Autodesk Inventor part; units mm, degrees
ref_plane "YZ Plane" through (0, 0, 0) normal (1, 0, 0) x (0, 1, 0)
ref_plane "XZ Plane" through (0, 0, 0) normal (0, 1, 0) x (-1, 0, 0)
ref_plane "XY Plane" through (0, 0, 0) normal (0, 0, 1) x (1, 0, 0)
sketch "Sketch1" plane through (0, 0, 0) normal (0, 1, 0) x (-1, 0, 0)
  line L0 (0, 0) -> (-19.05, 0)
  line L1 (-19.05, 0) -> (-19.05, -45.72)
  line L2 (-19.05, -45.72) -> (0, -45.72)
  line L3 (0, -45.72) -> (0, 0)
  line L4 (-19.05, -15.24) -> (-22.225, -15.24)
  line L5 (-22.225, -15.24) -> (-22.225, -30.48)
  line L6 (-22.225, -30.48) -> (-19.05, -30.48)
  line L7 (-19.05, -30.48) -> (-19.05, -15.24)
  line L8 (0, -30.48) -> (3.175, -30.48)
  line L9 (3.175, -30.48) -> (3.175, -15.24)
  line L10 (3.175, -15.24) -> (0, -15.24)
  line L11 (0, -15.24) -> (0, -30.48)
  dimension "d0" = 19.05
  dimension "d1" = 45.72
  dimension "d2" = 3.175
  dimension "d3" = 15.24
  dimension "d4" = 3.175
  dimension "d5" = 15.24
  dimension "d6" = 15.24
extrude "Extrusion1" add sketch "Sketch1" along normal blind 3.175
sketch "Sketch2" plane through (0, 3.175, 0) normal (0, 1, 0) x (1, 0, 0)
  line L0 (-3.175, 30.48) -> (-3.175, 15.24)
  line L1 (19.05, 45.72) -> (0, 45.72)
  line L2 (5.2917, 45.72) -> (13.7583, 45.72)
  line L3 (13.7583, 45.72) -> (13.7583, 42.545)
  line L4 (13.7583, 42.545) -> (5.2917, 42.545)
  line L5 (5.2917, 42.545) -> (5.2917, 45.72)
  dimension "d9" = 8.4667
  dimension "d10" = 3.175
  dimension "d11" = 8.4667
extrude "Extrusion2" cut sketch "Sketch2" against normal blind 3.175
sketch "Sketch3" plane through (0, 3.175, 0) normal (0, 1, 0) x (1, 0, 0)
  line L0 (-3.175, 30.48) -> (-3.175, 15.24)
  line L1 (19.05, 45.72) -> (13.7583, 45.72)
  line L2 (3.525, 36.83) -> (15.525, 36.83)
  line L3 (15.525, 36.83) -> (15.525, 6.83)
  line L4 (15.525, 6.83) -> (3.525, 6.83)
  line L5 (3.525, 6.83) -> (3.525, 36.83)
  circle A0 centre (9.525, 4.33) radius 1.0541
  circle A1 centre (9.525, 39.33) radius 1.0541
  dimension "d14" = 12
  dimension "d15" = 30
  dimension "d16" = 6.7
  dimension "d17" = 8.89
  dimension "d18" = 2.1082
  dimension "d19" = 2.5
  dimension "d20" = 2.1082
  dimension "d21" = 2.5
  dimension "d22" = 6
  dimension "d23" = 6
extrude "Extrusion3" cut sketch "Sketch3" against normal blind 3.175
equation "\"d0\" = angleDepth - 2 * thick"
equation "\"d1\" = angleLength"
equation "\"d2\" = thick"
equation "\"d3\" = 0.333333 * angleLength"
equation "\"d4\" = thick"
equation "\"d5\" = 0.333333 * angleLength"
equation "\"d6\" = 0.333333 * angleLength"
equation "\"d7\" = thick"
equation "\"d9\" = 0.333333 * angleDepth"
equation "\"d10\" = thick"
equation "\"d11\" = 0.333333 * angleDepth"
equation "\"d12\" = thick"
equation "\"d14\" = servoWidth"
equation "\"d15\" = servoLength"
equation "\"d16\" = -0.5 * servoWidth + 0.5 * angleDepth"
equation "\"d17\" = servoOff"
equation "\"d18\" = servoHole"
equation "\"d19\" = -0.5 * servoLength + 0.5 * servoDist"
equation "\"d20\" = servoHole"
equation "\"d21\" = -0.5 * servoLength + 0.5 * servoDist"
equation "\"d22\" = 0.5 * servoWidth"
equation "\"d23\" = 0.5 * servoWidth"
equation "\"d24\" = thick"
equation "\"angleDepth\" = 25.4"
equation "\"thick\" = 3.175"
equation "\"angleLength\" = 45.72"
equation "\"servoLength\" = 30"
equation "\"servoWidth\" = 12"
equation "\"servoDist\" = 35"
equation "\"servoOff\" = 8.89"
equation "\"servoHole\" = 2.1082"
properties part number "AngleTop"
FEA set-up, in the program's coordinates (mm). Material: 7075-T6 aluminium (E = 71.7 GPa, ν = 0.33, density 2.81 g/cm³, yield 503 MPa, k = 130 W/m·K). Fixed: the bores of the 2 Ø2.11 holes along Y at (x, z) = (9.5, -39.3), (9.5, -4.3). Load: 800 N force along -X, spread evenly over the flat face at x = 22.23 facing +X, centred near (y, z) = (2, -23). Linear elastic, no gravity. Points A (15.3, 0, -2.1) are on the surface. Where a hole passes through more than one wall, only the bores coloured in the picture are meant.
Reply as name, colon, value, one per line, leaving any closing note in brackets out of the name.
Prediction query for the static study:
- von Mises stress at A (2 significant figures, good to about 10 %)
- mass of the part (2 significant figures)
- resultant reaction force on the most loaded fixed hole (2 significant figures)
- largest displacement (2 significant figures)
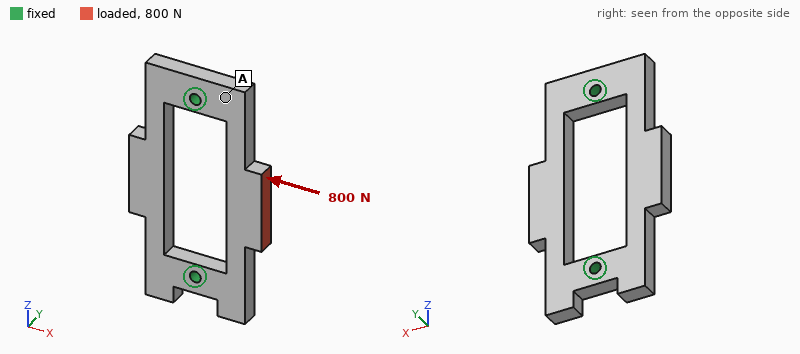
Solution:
von Mises stress at A: 26 MPa
mass of the part: 5.1 g
resultant reaction force on the most loaded fixed hole: 570 N
largest displacement: 87 µm
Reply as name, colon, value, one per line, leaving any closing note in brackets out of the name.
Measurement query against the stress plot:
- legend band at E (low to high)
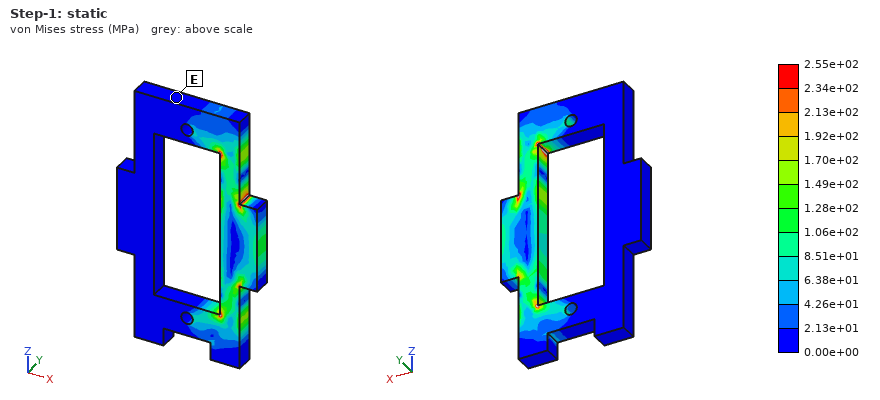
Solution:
legend band at E: 0.00e+00 to 2.13e+01 MPa
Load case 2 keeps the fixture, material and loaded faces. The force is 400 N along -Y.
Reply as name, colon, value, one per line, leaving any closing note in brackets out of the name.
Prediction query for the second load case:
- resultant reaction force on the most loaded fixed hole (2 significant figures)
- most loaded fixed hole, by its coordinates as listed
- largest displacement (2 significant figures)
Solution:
resultant reaction force on the most loaded fixed hole: 210 N
most loaded fixed hole, by its coordinates as listed: (9.5, -39.3)
largest displacement: 0.35 mm
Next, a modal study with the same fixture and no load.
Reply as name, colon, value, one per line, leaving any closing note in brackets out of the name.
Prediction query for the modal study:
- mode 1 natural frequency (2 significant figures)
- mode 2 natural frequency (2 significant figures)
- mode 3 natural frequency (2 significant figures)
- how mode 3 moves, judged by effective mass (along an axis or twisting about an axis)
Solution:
mode 1 natural frequency: 7100 Hz
mode 2 natural frequency: 7100 Hz
mode 3 natural frequency: 15 kHz
how mode 3 moves, judged by effective mass: along X
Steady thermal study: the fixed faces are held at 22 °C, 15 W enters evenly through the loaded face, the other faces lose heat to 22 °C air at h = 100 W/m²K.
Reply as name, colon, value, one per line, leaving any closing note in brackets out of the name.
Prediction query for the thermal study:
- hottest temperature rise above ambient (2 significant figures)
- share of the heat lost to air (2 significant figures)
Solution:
hottest temperature rise above ambient: 75 K
share of the heat lost to air: 20 %
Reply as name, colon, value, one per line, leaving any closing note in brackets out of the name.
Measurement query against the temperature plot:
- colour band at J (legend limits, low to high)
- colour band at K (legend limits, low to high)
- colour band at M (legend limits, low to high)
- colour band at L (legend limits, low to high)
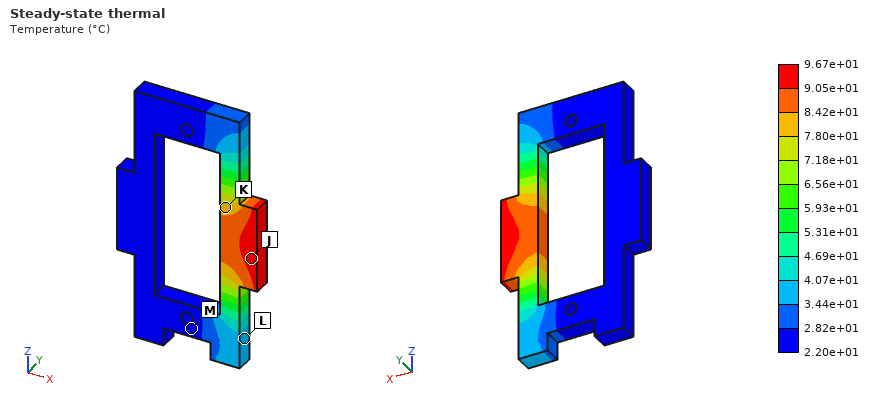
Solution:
colour band at J: 9.05e+01 to 9.67e+01 °C
colour band at K: 7.80e+01 to 8.42e+01 °C
colour band at M: 2.20e+01 to 2.82e+01 °C
colour band at L: 3.44e+01 to 4.07e+01 °C
